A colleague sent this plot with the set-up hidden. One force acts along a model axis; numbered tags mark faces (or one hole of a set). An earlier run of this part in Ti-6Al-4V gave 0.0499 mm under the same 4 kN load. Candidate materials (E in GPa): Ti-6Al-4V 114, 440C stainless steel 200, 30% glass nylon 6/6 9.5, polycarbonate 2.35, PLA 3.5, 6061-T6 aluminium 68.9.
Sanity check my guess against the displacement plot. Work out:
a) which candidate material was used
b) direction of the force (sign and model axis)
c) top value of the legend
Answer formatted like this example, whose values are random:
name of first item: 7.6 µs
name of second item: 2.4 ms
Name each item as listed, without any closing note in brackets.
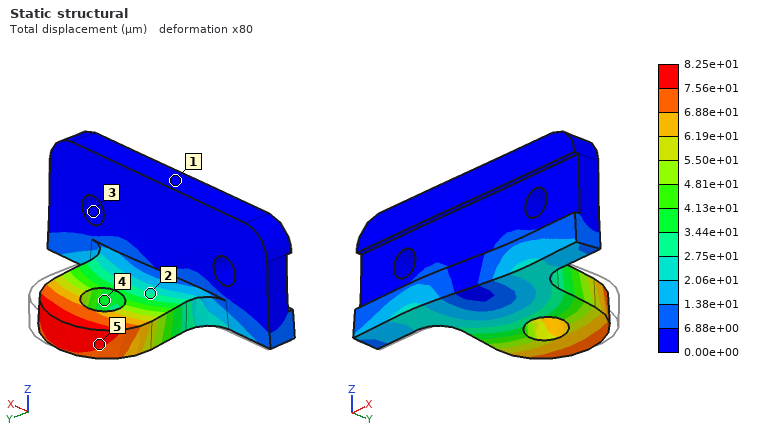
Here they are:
which candidate material was used: 6061-T6 aluminium
direction of the force: -X
top value of the legend: 8.25e+01 µm
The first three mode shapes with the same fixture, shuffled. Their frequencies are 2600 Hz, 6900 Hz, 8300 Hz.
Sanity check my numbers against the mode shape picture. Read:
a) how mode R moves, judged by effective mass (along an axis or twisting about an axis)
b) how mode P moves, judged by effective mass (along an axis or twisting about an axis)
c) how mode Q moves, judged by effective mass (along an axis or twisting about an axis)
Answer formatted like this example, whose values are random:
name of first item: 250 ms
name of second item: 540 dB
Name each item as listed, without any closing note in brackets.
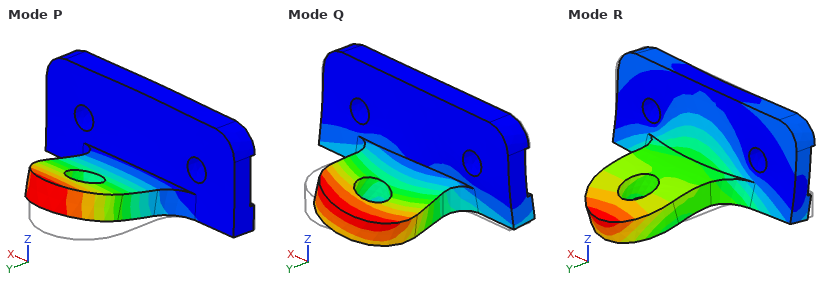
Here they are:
how mode R moves, judged by effective mass: along Y
how mode P moves, judged by effective mass: along Z
how mode Q moves, judged by effective mass: along X
